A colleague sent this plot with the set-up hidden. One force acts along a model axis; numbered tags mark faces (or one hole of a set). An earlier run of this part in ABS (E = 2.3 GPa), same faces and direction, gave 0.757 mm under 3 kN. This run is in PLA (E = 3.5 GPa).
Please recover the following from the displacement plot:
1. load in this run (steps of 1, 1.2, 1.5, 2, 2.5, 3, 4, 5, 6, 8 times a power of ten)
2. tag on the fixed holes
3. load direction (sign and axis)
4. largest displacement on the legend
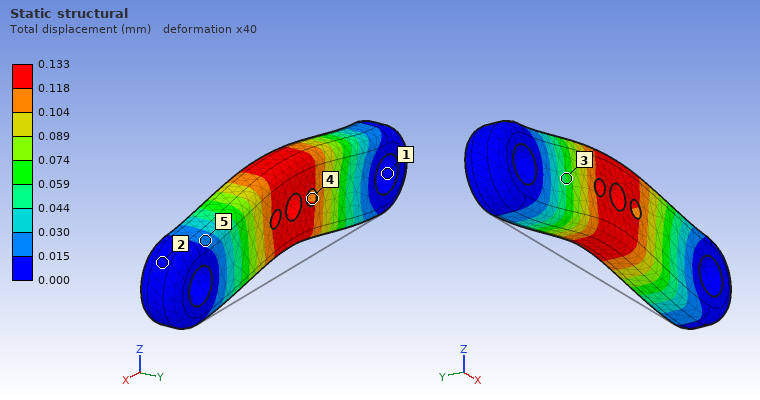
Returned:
800 N
1
+Z
0.133 mm
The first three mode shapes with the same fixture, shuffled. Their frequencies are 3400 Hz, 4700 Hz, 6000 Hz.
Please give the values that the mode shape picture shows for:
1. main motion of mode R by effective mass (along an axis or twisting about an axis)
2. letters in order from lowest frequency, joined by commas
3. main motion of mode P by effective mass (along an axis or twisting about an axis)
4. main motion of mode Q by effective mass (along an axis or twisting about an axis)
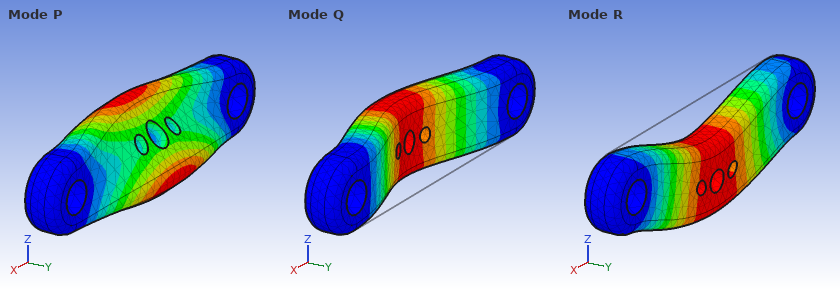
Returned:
along Z
Q, R, P
twisting about X
along Y
